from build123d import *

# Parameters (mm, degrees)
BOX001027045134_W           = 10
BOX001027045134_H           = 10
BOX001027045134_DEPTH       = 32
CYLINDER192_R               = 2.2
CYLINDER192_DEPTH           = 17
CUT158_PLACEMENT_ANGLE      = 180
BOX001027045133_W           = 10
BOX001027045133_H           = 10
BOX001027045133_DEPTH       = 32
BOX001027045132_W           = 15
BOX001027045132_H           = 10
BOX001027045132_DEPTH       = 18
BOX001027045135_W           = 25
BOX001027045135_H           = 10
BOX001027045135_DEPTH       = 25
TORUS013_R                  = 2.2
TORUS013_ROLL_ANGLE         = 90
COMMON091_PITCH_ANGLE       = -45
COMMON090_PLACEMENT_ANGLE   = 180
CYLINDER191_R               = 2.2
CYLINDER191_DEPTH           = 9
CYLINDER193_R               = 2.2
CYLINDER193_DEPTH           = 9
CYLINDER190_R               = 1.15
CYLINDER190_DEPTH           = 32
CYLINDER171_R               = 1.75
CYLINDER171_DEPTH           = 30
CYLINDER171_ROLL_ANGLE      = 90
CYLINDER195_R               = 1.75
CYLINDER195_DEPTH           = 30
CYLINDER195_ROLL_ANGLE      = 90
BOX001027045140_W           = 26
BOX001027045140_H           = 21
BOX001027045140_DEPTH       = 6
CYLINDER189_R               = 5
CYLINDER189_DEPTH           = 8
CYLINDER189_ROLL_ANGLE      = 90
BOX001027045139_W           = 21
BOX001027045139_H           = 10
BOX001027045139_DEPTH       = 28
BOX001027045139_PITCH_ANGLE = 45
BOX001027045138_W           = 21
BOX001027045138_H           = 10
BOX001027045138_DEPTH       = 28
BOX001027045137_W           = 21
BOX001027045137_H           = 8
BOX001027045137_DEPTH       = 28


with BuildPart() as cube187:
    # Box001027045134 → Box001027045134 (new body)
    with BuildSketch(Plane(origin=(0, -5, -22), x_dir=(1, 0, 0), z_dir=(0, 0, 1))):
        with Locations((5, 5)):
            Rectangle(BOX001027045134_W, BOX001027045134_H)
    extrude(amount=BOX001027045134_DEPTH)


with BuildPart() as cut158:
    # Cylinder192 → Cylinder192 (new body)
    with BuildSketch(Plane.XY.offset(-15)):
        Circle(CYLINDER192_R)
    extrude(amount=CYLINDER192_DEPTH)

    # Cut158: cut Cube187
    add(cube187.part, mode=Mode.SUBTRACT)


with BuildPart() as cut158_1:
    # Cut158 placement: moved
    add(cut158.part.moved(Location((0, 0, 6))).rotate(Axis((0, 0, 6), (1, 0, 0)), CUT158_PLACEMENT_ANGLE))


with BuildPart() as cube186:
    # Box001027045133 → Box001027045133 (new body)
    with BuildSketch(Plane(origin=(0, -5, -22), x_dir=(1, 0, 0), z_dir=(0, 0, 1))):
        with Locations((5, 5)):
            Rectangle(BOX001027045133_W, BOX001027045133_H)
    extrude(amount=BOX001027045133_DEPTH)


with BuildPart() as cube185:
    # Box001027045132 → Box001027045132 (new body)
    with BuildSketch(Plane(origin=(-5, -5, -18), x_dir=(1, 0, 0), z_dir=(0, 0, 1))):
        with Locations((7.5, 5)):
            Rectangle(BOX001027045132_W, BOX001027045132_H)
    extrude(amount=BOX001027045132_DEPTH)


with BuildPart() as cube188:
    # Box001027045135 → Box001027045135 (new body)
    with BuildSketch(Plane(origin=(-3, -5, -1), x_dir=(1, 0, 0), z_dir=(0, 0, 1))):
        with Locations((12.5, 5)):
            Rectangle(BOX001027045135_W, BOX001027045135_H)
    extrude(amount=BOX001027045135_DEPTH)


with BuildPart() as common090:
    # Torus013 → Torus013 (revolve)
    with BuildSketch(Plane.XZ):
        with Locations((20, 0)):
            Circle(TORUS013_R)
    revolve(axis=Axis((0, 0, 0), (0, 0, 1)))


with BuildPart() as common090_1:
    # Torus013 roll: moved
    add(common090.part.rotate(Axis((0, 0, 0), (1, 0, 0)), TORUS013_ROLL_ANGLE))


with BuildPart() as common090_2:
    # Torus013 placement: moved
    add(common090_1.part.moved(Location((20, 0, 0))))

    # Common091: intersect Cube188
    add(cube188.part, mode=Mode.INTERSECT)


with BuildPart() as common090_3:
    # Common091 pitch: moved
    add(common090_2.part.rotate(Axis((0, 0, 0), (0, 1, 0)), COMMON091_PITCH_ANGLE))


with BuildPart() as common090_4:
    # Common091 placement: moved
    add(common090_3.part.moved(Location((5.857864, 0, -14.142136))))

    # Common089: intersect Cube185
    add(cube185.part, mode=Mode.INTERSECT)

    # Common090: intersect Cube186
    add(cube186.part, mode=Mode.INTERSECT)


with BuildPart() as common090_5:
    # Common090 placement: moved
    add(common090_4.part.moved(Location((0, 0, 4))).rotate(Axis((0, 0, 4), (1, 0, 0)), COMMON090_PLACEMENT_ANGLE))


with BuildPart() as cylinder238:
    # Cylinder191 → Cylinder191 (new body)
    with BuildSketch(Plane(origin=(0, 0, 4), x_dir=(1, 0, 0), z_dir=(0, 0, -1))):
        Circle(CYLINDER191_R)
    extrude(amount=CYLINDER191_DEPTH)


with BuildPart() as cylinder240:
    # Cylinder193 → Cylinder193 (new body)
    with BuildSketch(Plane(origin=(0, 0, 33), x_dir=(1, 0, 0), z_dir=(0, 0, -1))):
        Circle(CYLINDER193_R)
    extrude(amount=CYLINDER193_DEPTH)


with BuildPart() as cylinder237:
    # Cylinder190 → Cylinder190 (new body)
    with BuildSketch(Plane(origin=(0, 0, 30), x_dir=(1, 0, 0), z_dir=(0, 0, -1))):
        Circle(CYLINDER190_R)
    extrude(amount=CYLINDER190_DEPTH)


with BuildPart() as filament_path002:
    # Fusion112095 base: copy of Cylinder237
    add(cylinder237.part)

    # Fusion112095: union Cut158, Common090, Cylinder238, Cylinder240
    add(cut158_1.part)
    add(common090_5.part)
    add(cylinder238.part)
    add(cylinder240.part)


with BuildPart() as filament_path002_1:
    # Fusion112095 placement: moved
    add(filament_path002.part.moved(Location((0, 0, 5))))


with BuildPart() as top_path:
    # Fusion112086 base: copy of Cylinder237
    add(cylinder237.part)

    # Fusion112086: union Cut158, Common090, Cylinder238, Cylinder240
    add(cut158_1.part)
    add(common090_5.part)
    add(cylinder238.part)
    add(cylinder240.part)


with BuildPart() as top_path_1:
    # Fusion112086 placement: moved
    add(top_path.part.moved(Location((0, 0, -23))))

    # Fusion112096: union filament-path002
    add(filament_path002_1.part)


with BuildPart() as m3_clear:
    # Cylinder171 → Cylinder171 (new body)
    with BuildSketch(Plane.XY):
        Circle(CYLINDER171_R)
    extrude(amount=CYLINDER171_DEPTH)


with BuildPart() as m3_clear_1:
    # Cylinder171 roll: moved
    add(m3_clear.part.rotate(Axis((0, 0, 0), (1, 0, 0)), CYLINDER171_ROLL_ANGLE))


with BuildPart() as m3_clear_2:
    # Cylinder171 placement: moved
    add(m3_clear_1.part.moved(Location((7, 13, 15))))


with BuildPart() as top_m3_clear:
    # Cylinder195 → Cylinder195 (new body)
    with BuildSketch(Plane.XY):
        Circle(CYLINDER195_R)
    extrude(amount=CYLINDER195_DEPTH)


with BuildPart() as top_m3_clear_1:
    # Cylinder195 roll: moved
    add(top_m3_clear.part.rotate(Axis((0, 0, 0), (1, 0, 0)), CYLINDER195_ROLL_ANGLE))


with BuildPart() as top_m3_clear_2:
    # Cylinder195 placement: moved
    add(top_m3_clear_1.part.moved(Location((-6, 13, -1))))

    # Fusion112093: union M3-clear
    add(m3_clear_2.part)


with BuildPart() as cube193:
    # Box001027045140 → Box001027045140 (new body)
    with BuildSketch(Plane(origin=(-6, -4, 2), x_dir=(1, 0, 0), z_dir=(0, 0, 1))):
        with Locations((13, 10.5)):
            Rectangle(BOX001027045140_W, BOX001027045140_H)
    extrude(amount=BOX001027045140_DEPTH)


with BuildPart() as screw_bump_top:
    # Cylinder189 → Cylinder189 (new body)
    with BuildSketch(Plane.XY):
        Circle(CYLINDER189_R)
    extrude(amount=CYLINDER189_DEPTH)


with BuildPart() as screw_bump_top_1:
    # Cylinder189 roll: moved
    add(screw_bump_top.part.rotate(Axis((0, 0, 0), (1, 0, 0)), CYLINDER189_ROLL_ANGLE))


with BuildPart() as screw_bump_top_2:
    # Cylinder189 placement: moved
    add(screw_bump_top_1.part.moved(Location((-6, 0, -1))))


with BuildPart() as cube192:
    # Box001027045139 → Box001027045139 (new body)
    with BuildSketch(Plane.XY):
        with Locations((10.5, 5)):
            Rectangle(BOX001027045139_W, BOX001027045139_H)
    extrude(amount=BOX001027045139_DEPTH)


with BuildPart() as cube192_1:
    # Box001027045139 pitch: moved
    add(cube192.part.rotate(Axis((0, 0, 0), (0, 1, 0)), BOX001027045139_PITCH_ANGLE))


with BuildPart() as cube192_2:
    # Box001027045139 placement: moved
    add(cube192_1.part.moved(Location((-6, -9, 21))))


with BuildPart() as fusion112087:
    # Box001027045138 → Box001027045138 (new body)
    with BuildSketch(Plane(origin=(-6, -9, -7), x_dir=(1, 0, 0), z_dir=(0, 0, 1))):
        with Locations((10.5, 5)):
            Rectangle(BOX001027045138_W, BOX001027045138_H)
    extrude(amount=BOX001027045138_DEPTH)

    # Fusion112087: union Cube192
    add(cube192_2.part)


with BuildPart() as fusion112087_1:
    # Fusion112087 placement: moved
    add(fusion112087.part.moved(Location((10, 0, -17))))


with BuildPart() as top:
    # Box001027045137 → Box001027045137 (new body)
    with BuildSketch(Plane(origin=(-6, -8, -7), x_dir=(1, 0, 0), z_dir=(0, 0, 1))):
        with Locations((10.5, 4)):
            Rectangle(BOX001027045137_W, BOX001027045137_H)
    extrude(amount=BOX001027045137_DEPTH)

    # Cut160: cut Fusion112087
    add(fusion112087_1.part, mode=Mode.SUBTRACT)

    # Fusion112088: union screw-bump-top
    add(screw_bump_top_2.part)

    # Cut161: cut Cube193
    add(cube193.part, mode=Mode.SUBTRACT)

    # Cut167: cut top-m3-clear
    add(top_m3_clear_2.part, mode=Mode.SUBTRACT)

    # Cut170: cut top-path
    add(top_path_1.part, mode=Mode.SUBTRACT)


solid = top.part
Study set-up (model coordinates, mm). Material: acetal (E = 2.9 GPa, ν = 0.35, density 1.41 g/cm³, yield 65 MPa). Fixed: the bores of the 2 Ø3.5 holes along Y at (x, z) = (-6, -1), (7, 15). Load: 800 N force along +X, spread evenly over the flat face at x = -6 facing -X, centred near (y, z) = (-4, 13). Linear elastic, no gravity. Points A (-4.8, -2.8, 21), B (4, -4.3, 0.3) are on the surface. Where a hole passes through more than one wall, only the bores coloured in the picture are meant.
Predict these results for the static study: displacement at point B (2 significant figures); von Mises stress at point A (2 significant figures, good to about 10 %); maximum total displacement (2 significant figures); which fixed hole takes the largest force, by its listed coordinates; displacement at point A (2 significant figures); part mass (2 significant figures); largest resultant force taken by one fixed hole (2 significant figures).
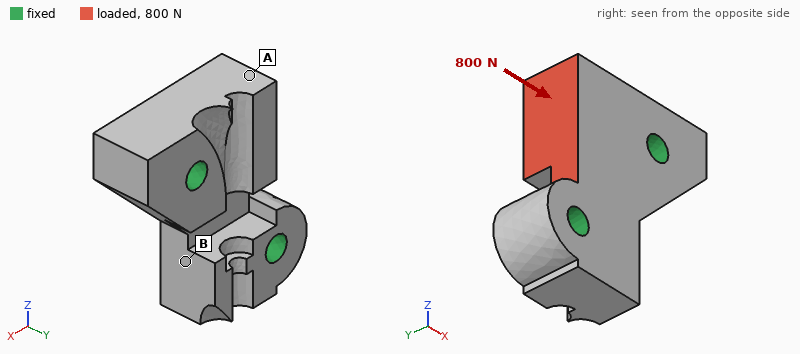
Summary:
15 µm
8.7 MPa
88 µm
(7, 15)
61 µm
4.2 g
690 N
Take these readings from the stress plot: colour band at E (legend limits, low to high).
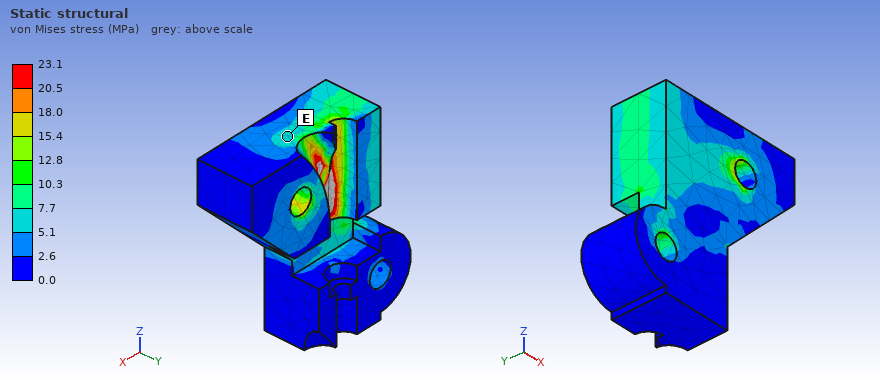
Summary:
5.1 to 7.7 MPa
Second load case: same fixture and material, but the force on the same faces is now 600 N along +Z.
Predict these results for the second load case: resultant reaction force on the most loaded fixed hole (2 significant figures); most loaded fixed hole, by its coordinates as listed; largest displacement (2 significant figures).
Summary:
400 N
(-6, -1)
0.17 mm
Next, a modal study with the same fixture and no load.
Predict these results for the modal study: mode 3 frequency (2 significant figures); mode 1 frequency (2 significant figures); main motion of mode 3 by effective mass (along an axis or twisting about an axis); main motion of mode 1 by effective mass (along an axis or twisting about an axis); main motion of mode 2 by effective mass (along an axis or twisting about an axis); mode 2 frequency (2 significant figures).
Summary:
14 kHz
8500 Hz
along Y
along Y
along Z
12 kHz
